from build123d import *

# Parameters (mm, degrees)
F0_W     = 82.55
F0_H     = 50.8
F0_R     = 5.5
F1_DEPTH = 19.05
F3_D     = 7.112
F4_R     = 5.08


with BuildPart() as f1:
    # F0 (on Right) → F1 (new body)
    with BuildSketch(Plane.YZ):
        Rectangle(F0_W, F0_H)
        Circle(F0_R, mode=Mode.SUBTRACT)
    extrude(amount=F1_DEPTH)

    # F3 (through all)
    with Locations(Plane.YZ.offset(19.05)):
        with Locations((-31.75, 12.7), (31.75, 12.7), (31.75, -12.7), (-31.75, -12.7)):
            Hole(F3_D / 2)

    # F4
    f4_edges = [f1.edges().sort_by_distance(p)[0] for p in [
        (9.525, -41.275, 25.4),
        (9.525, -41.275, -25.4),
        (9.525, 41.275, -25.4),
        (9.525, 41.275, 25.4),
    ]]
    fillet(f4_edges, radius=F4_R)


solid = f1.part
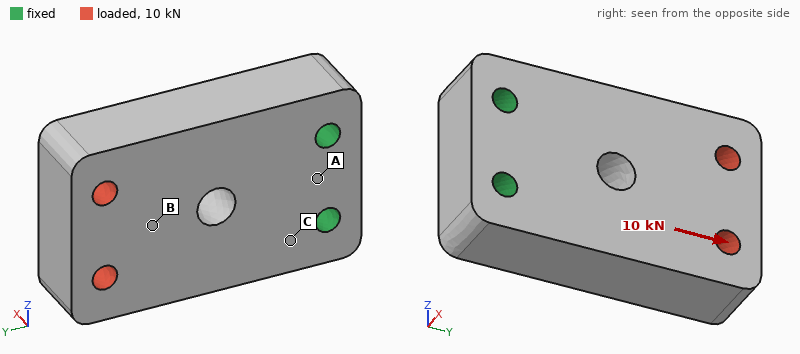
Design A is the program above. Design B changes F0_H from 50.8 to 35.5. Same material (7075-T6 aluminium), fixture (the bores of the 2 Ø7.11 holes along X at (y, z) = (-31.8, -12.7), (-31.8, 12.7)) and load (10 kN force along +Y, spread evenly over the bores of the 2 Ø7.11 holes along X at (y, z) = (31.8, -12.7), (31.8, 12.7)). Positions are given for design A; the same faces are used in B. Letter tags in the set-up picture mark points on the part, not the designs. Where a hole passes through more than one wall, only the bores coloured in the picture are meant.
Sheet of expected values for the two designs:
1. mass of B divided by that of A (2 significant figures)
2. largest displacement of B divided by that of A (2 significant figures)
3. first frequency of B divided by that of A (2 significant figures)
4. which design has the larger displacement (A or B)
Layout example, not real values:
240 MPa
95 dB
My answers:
0.68
1.5
1.0
B
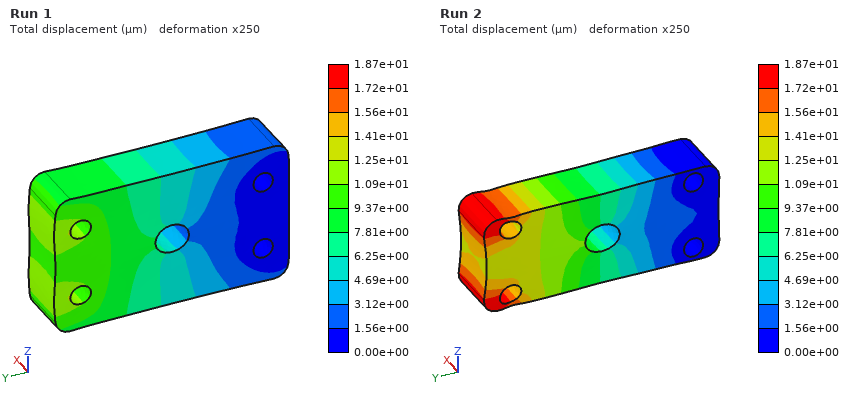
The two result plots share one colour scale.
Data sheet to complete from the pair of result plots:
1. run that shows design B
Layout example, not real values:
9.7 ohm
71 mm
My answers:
Run 2
